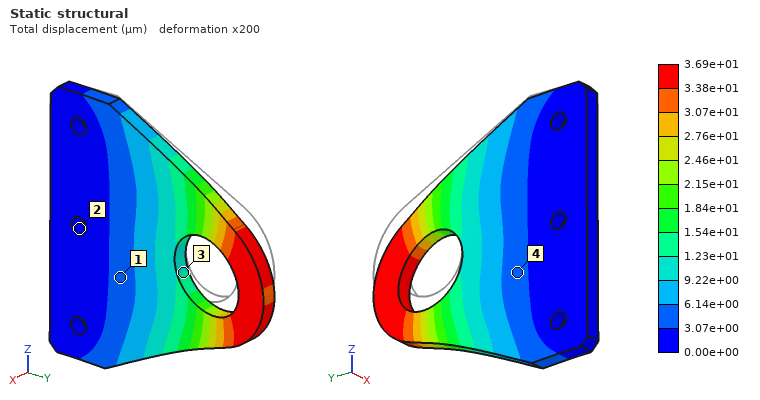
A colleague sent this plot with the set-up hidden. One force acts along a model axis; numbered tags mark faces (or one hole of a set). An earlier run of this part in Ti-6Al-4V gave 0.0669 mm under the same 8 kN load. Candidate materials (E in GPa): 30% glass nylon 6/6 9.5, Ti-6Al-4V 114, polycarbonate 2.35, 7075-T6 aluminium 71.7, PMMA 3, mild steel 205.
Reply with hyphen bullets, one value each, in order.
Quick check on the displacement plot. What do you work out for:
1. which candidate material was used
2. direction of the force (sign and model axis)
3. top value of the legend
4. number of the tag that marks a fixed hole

- mild steel
- -Z
- 3.69e+01 µm
- 2
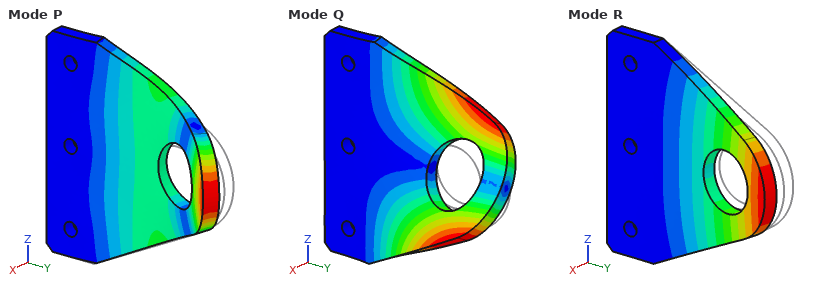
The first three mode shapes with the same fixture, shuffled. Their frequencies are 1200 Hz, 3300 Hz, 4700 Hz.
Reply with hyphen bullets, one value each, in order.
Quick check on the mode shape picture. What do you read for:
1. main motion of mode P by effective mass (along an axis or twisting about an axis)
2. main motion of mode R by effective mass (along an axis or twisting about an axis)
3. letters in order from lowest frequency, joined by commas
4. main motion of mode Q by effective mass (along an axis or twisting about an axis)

- along X
- along X
- R, Q, P
- twisting about Y
